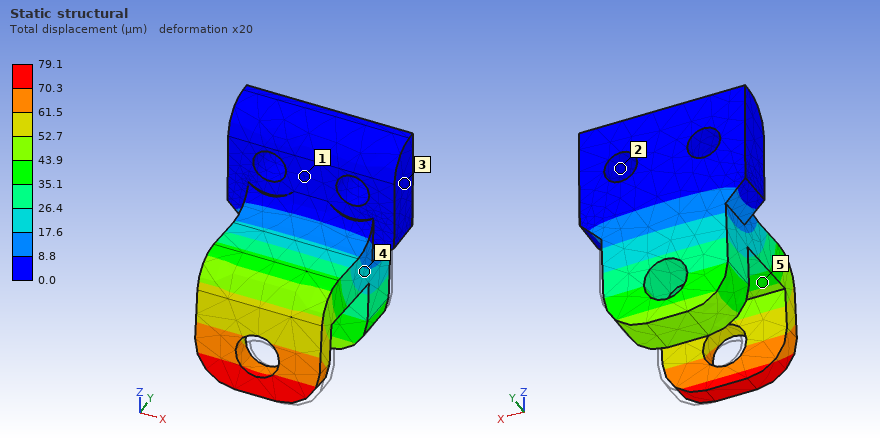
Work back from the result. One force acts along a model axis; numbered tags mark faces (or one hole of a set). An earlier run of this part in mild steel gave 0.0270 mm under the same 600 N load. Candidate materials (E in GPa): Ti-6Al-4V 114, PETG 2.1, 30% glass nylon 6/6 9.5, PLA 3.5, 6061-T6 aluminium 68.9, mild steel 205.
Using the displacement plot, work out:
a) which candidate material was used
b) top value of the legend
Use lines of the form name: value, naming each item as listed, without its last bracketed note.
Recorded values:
which candidate material was used: 6061-T6 aluminium
top value of the legend: 79.1 µm
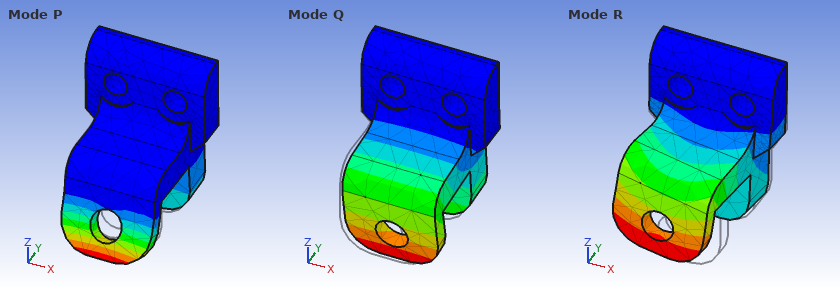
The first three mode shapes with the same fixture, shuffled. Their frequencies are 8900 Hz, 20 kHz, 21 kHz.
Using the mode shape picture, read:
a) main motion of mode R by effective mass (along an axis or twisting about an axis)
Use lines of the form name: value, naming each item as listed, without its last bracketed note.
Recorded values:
main motion of mode R by effective mass: along X
